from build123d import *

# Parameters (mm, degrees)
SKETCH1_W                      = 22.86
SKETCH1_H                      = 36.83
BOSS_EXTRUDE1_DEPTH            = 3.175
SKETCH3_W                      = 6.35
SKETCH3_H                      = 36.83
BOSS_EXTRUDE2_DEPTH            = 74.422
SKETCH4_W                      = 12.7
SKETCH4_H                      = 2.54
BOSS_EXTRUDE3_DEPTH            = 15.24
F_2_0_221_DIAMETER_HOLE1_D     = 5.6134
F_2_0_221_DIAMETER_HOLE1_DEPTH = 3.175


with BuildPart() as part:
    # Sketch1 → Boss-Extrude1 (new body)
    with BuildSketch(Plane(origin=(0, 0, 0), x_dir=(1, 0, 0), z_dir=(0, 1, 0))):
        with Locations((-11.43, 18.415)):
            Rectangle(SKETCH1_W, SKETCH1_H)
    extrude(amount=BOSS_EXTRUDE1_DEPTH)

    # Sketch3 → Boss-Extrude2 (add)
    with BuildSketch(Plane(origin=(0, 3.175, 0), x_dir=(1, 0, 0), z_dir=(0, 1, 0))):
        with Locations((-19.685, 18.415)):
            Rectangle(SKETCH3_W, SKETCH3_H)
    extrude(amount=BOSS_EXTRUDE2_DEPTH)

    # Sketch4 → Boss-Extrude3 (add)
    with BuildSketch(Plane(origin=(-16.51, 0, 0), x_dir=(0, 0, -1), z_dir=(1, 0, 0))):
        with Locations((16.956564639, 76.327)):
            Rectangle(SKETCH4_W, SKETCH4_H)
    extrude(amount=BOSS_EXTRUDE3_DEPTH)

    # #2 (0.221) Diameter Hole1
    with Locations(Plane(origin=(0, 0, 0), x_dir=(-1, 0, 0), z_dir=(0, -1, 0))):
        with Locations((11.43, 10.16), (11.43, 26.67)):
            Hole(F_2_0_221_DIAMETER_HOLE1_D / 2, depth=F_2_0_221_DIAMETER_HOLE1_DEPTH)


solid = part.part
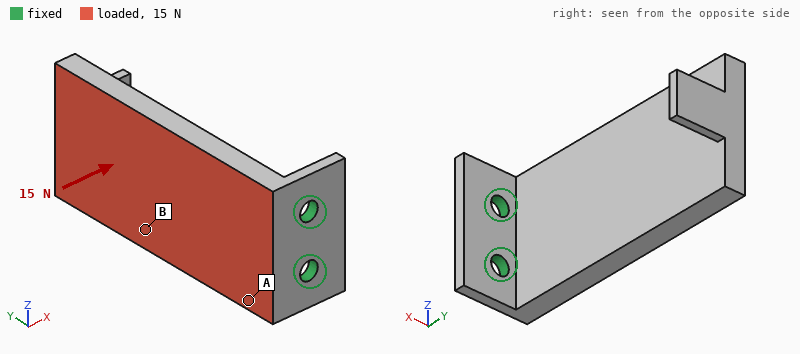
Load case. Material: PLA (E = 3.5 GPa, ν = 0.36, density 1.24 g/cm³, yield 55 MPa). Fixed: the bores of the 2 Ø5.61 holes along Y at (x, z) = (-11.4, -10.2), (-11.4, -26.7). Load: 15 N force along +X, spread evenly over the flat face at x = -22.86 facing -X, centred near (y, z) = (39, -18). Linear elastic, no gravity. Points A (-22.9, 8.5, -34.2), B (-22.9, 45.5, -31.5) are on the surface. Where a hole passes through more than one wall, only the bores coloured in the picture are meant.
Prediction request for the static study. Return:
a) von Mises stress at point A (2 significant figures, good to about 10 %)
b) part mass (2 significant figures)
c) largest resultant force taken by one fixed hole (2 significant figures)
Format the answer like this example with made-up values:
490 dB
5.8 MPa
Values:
1.9 MPa
25 g
8.3 N
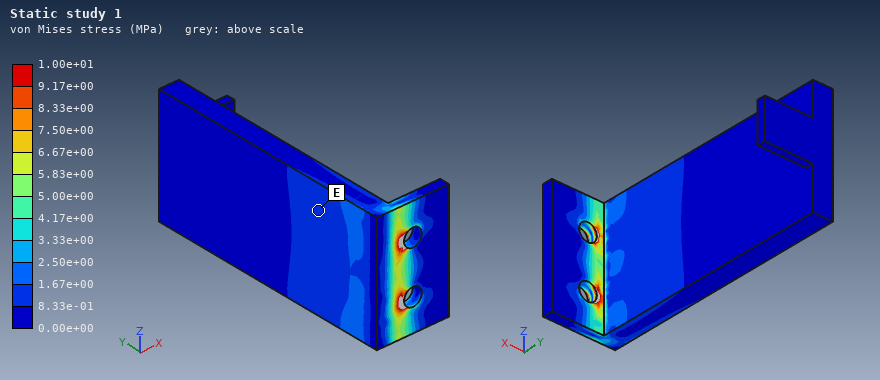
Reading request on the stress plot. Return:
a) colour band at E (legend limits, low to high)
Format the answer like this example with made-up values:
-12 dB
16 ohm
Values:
8.33e-01 to 1.67e+00 MPa
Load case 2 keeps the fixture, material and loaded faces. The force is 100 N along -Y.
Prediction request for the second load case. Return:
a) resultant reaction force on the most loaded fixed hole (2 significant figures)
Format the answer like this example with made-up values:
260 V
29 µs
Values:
50 N
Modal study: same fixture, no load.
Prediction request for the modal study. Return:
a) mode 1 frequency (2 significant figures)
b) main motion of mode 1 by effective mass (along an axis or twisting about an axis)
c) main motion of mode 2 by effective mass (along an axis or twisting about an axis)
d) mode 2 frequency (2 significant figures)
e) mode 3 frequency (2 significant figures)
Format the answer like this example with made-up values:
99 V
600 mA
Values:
160 Hz
along X
along Z
560 Hz
1100 Hz
